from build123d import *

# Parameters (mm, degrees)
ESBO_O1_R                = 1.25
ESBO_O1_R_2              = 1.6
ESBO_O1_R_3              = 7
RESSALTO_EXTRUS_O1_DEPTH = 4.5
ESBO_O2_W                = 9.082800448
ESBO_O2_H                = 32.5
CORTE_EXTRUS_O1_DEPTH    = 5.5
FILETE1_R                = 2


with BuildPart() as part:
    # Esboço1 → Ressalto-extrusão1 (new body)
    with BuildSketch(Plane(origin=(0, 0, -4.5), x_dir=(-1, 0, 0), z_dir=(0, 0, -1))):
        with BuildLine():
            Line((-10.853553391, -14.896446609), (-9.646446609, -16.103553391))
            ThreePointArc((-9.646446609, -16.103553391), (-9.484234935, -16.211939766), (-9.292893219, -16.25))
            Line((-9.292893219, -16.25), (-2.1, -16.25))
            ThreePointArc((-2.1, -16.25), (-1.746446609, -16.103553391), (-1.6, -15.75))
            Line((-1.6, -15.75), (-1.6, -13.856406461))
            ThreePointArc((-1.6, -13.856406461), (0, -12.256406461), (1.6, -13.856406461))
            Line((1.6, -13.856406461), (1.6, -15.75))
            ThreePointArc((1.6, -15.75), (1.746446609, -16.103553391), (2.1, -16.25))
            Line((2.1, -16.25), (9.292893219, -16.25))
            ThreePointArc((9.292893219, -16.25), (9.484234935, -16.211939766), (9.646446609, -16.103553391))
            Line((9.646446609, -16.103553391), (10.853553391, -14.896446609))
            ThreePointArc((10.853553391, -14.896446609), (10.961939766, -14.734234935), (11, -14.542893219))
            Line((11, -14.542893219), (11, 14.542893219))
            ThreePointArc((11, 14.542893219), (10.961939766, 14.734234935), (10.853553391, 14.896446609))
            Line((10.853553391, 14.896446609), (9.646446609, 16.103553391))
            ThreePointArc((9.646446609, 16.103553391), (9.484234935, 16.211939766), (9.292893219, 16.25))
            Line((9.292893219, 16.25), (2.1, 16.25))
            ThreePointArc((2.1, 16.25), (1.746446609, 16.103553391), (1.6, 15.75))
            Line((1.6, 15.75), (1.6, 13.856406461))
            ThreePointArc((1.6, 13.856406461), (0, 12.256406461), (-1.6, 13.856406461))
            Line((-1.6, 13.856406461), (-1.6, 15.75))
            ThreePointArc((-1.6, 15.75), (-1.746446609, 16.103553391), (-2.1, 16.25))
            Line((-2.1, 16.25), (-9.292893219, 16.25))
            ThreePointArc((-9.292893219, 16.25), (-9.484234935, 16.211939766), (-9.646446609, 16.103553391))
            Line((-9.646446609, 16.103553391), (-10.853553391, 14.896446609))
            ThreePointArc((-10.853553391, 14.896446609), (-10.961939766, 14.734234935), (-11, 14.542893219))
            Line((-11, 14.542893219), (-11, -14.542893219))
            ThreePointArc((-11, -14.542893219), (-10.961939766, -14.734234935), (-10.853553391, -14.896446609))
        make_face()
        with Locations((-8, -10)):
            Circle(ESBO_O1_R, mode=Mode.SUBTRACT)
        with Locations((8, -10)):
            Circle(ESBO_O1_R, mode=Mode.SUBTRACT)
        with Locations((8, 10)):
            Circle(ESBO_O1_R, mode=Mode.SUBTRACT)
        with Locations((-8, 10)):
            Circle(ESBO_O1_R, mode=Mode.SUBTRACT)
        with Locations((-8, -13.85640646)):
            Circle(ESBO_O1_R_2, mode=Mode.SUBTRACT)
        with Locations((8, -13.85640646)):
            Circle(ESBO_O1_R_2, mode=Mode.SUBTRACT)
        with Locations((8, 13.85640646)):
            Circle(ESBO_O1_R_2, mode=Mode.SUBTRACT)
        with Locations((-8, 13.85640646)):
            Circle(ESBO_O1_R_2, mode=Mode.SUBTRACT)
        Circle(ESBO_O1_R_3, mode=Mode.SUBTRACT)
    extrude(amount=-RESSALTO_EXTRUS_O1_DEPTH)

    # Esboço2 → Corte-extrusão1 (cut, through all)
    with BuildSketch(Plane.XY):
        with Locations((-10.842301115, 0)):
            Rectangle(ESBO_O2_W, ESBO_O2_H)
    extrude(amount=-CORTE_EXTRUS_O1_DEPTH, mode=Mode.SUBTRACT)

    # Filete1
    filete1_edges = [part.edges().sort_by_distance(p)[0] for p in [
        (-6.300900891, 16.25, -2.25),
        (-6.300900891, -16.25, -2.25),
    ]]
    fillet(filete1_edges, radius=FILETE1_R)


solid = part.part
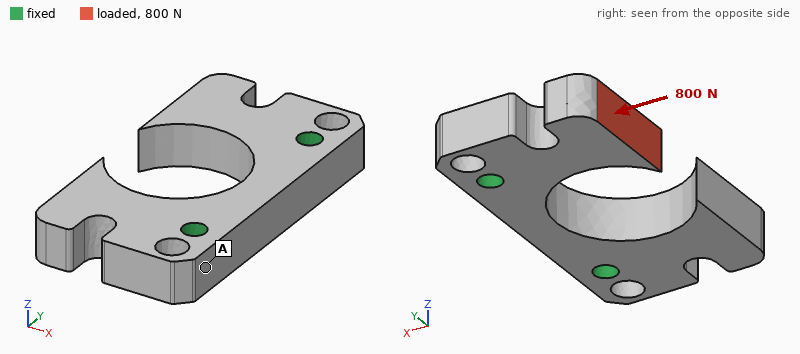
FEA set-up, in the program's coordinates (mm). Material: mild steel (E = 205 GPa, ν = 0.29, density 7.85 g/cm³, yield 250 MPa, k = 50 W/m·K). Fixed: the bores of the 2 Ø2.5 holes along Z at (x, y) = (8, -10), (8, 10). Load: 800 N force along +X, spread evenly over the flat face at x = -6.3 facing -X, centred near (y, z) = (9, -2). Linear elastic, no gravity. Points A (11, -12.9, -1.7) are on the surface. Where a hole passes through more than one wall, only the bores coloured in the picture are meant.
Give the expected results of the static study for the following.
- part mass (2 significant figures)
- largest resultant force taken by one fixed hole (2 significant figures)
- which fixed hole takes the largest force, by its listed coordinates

13 g
760 N
(8, 10)
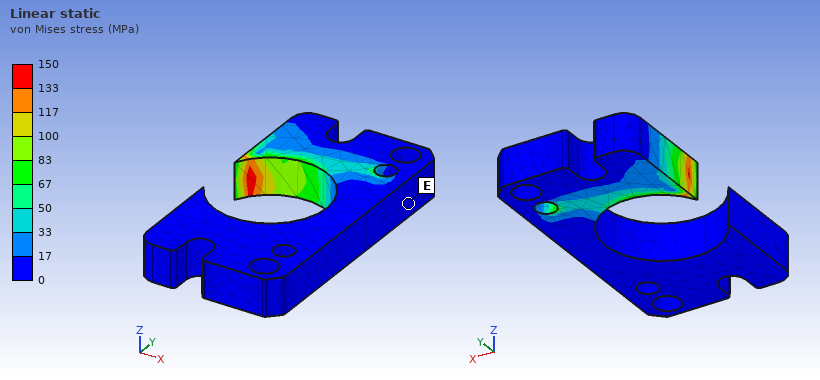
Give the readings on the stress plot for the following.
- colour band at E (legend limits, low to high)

0 to 17 MPa
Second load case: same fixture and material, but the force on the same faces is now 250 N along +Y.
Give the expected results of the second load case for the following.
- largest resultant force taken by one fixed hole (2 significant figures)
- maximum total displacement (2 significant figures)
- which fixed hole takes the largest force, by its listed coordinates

280 N
18 µm
(8, 10)
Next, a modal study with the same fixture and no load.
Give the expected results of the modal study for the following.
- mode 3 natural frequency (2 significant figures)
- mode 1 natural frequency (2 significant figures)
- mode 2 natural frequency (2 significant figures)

17 kHz
15 kHz
15 kHz
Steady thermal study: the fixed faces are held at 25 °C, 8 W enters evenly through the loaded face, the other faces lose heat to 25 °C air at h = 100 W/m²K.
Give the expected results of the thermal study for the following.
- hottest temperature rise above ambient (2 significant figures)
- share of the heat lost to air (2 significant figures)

81 K
18 %
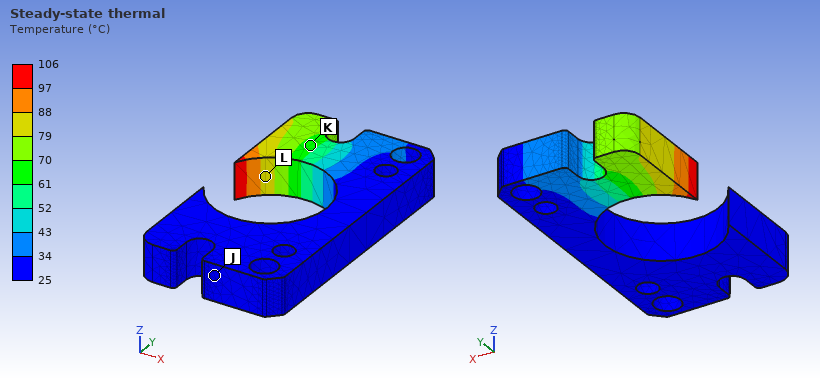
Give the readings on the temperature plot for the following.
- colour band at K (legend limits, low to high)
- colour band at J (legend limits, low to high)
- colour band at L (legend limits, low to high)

61 to 70 °C
25 to 34 °C
79 to 88 °C
